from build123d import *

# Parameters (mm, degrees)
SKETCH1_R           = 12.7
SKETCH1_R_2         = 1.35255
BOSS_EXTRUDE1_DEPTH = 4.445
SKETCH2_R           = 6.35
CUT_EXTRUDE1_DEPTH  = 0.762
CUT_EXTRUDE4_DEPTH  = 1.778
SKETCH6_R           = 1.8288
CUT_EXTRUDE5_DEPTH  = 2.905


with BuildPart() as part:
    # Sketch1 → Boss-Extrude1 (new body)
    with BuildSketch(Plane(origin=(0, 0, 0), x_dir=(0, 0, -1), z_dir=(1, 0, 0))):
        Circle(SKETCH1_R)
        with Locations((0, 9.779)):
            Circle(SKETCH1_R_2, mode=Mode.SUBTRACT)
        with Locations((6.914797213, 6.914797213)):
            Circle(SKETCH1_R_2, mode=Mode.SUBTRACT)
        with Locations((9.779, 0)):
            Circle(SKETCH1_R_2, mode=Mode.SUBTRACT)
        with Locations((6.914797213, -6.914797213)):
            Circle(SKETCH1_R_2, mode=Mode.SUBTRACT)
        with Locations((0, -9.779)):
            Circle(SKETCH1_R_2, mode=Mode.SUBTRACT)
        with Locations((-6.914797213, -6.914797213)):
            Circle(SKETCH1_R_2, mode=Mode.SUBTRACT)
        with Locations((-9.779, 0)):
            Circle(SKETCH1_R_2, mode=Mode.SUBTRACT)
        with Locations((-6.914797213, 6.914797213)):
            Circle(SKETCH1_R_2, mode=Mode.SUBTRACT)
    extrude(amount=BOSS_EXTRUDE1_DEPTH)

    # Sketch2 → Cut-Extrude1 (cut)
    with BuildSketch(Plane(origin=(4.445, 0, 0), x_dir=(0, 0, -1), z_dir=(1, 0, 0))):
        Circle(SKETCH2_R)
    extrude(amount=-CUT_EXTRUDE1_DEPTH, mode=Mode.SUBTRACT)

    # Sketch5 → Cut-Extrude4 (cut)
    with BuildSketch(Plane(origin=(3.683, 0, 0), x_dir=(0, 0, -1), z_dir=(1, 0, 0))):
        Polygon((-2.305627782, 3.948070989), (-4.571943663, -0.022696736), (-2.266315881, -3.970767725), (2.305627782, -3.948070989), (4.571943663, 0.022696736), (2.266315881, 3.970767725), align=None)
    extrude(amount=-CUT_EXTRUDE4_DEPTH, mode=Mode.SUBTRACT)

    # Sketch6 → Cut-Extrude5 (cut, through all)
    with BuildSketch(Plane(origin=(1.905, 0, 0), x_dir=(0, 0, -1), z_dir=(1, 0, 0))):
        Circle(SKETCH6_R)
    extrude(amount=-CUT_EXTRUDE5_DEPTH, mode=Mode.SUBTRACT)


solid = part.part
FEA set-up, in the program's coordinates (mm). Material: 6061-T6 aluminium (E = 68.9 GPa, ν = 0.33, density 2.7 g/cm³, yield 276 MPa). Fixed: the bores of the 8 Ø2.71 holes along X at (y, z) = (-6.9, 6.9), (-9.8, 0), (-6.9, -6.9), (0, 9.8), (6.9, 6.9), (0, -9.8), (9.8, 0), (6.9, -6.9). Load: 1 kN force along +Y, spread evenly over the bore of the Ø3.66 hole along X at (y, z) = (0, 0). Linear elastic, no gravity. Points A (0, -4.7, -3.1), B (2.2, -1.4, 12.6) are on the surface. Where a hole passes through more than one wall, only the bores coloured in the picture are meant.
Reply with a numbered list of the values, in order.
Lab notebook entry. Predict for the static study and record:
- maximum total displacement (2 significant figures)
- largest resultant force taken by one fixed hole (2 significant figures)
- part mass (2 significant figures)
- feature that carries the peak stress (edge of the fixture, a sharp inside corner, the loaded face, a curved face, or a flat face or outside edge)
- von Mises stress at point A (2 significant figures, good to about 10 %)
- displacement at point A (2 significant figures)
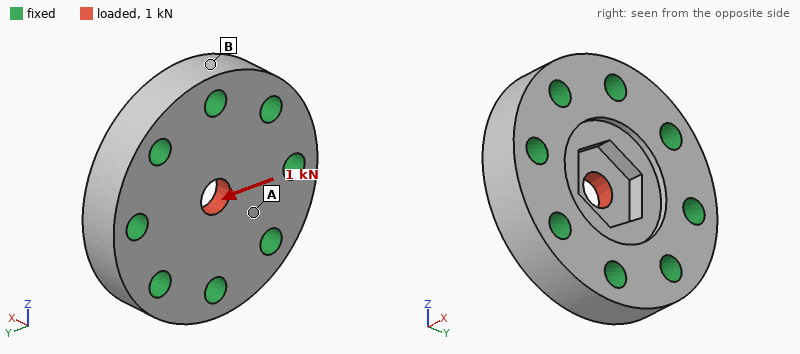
1. 2.9 µm
2. 230 N
3. 5.0 g
4. the loaded face
5. 18 MPa
6. 0.87 µm
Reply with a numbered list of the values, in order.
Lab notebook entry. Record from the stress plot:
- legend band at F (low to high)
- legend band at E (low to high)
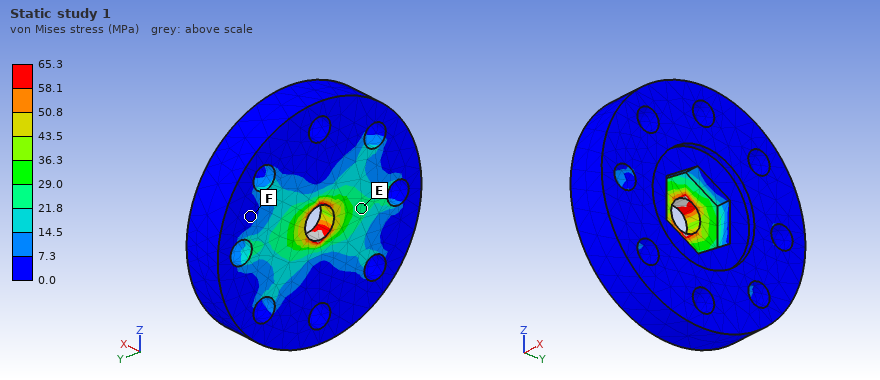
1. 0.0 to 7.3 MPa
2. 21.8 to 29.0 MPa
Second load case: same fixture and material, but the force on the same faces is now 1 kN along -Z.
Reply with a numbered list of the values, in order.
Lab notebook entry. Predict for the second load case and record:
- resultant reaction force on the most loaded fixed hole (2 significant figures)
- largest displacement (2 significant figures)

1. 230 N
2. 3.0 µm
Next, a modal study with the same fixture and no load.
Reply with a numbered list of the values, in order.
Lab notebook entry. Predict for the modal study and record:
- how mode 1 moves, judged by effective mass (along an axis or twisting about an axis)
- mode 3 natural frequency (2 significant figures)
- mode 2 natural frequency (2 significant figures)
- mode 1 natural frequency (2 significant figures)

1. along X
2. 130 kHz
3. 130 kHz
4. 100 kHz
